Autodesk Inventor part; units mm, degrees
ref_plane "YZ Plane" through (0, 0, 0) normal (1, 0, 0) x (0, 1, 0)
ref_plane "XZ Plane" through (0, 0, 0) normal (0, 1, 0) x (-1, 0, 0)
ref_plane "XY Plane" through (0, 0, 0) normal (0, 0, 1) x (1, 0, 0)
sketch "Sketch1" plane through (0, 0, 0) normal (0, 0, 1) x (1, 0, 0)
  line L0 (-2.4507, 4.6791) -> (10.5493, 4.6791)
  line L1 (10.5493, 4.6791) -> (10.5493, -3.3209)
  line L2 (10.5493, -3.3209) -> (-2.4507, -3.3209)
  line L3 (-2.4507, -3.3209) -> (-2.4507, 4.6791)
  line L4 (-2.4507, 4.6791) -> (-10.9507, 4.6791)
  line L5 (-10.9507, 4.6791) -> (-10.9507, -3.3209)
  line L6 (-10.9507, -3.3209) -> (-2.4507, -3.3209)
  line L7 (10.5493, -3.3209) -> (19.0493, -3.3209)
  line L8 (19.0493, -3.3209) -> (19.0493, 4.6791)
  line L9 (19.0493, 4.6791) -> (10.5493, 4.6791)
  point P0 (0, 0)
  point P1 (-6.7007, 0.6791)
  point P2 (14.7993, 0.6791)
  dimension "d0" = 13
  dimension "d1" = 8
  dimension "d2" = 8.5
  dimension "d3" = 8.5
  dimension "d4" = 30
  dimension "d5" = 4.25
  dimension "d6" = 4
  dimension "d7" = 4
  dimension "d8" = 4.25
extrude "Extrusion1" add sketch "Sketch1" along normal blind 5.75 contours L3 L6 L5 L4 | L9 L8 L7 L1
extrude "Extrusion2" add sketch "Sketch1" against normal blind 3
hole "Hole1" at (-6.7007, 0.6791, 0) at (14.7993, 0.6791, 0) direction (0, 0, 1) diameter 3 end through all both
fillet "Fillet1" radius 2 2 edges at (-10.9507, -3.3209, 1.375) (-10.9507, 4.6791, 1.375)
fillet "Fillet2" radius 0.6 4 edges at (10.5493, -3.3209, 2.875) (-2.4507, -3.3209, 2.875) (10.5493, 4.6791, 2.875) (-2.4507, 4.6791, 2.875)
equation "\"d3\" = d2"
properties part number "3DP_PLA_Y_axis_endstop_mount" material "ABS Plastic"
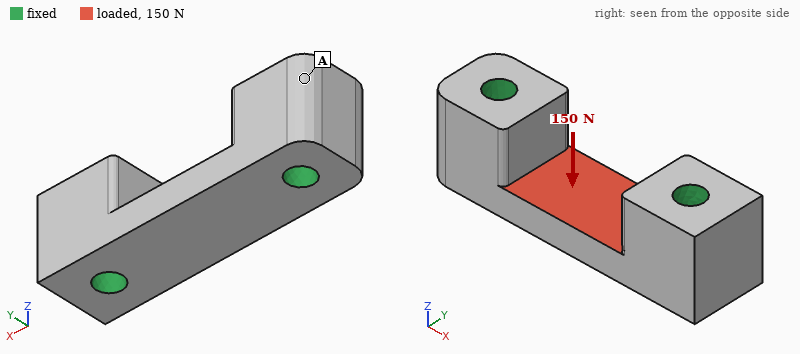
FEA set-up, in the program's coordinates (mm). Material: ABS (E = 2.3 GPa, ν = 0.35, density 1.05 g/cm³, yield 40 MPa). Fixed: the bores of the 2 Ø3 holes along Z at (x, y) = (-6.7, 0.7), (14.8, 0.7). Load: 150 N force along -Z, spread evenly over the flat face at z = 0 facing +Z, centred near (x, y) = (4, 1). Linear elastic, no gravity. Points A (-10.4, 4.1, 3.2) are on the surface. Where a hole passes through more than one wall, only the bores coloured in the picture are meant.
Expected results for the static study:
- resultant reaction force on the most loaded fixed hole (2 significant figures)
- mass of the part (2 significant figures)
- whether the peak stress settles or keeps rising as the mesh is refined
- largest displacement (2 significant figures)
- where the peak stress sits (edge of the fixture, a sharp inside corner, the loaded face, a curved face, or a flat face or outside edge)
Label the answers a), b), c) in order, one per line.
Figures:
a) 77 N
b) 1.4 g
c) keeps rising
d) 70 µm
e) a sharp inside corner
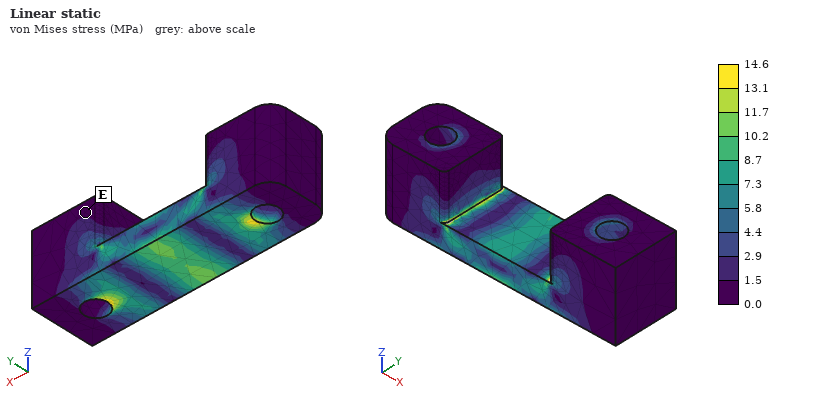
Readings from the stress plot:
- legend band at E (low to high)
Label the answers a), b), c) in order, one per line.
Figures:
a) 0.0 to 1.5 MPa
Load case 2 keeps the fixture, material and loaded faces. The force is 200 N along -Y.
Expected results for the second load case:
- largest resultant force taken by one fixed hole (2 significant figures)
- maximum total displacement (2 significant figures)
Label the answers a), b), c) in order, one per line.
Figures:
a) 100 N
b) 86 µm
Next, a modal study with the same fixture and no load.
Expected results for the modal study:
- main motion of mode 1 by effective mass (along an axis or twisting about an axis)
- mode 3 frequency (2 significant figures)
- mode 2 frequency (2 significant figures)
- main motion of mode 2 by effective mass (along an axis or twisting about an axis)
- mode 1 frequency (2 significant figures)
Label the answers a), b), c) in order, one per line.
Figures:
a) along Z
b) 20 kHz
c) 17 kHz
d) along Y
e) 15 kHz
